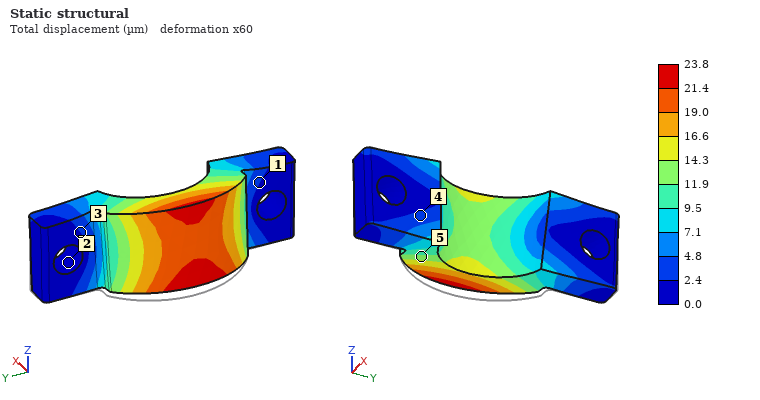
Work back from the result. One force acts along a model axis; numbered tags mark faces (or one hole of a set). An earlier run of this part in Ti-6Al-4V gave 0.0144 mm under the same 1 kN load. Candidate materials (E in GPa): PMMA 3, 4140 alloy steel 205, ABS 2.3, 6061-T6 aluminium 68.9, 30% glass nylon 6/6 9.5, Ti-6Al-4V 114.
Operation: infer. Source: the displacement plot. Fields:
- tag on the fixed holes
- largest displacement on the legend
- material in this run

2
23.8 µm
6061-T6 aluminium
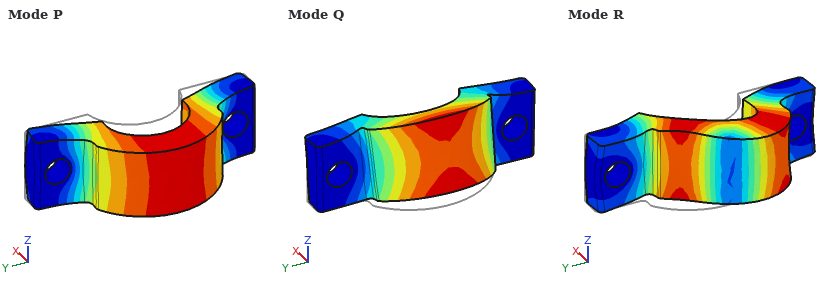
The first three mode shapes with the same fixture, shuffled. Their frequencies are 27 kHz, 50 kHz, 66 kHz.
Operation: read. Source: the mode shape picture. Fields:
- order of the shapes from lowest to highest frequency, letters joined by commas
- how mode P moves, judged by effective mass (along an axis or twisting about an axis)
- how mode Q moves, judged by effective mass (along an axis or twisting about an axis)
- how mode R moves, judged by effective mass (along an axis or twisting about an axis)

Q, P, R
along X
along Z
along Y
